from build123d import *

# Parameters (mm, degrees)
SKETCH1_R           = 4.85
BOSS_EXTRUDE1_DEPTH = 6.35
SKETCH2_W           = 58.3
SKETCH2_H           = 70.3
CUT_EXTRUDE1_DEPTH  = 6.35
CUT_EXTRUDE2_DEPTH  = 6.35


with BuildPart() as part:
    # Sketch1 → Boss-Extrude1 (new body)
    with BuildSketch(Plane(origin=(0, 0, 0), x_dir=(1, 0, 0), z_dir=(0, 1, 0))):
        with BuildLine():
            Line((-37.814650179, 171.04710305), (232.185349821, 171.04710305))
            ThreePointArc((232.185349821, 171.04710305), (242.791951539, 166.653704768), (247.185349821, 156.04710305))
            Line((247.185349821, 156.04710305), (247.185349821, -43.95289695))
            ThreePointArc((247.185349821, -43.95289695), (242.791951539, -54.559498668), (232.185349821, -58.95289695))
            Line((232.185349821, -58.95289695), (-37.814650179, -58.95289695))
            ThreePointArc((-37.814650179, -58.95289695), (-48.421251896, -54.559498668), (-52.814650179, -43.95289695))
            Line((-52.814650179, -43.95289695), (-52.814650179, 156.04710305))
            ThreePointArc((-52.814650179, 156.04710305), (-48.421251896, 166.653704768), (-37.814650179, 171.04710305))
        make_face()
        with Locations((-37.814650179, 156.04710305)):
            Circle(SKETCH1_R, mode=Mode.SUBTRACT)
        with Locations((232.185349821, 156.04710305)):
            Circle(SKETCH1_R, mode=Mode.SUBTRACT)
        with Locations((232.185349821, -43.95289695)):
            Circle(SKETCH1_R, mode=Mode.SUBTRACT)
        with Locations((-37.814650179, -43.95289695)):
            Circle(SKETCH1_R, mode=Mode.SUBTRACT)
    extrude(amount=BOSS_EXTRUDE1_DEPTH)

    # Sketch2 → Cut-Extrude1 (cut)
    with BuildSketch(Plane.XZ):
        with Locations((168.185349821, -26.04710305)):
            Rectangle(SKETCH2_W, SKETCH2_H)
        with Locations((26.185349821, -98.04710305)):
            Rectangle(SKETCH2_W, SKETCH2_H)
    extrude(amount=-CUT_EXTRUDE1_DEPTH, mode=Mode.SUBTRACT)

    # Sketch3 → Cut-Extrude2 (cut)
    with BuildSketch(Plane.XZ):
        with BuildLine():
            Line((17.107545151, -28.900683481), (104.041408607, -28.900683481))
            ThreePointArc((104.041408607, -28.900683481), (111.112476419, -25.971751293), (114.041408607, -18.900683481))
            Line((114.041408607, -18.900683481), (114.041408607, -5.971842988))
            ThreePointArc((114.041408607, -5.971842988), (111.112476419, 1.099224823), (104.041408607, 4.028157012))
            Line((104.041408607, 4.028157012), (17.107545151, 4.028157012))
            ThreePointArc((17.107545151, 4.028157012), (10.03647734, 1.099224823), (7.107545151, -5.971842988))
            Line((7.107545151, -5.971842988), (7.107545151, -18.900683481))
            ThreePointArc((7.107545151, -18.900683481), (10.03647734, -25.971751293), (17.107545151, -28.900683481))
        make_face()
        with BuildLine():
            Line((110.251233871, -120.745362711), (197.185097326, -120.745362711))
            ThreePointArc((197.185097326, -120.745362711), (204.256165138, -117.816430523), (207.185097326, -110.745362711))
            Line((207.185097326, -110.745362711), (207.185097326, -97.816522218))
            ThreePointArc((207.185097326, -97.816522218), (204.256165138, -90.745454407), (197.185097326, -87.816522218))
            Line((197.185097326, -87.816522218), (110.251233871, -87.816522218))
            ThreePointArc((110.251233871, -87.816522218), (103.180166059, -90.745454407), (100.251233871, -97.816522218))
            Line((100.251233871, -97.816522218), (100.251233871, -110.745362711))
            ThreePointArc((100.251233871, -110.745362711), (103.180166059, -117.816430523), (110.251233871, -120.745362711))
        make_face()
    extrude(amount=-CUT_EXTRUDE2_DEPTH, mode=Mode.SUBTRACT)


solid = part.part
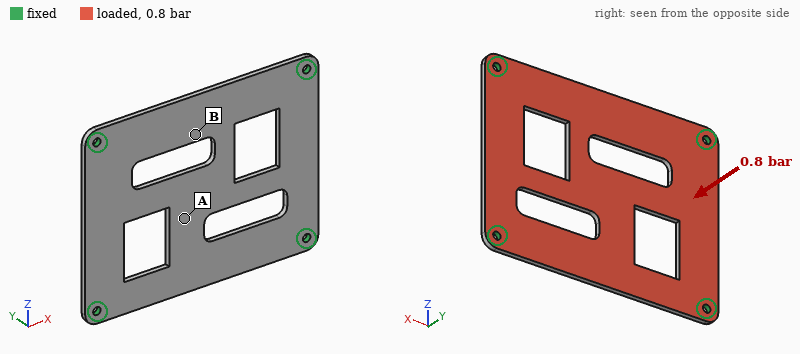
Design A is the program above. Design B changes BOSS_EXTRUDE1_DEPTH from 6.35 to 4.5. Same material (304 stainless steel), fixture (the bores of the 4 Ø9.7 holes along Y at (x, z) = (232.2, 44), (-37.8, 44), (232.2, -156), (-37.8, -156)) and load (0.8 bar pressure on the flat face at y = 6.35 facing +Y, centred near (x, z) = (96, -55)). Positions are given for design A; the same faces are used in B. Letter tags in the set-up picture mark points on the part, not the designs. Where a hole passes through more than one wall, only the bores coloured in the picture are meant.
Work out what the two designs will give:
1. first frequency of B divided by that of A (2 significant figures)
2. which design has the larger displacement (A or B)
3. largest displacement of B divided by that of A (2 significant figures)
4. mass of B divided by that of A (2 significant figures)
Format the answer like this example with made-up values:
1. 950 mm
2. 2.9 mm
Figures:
1. 0.72
2. B
3. 2.7
4. 0.71
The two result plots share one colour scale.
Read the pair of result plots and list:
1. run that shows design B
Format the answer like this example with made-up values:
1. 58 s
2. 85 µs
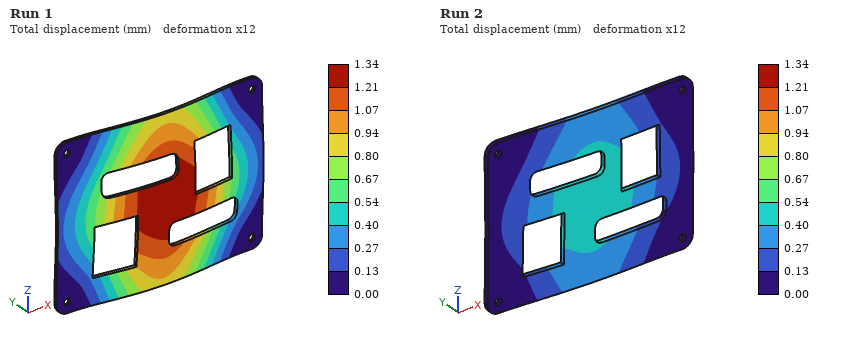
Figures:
1. Run 1
